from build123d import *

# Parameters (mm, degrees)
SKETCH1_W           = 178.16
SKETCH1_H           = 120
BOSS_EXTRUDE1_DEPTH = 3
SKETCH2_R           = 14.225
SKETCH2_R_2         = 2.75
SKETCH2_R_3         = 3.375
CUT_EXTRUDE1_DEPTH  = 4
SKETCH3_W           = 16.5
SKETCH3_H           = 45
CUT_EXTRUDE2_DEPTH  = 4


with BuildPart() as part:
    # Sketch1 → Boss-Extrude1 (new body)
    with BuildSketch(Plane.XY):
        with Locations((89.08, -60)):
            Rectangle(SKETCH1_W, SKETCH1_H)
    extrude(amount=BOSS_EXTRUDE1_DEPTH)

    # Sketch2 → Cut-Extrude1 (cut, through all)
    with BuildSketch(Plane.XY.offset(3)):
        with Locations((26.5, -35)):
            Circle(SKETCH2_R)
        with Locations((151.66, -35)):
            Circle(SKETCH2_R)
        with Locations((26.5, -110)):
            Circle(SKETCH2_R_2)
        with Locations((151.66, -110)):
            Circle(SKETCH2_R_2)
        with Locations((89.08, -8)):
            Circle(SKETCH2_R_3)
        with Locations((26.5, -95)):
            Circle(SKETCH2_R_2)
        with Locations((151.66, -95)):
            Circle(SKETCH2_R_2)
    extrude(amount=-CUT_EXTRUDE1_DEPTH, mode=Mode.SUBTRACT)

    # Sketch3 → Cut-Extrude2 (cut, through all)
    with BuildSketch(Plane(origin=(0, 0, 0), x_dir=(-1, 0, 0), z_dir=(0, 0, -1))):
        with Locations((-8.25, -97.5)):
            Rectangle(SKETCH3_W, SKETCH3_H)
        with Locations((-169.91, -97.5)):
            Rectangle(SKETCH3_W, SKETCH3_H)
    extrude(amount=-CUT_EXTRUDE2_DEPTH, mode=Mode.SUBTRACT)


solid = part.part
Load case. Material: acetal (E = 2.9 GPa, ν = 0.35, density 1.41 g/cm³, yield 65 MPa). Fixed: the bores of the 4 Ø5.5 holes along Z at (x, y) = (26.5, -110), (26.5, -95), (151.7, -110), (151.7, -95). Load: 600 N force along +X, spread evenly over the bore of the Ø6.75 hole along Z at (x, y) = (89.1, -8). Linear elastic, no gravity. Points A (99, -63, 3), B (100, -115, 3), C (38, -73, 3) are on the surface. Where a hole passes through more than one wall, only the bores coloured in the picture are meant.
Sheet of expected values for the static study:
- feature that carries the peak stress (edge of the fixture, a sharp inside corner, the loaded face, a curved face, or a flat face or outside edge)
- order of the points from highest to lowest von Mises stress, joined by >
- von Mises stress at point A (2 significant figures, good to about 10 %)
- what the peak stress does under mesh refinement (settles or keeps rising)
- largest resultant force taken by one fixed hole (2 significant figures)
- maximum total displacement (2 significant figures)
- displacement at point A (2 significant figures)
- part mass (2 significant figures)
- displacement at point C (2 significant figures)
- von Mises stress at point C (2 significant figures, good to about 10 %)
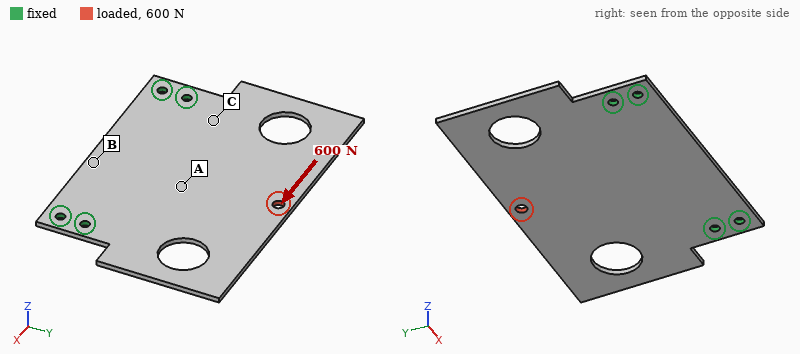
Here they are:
edge of the fixture
C > A > B
2.4 MPa
keeps rising
380 N
0.28 mm
0.077 mm
78 g
0.060 mm
4.6 MPa
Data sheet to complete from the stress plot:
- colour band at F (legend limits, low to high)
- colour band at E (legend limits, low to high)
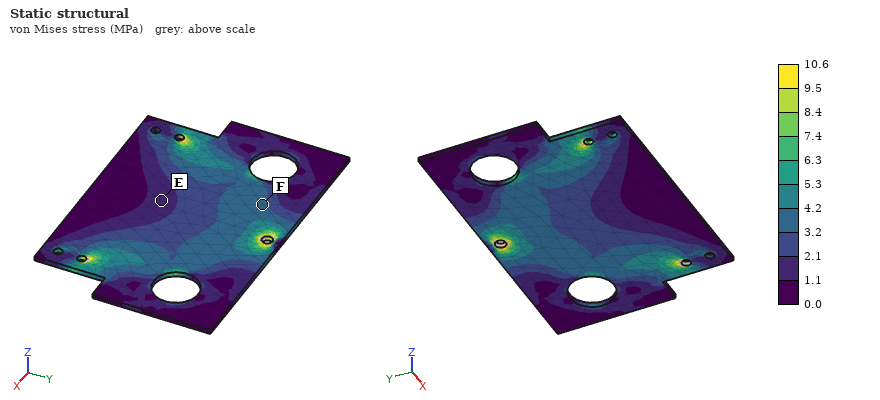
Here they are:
3.2 to 4.2 MPa
1.1 to 2.1 MPa
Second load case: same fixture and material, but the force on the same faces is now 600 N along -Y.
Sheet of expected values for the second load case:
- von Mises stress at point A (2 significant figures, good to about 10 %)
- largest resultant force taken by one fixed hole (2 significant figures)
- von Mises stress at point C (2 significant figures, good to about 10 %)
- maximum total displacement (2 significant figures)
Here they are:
1.6 MPa
210 N
2.8 MPa
0.19 mm
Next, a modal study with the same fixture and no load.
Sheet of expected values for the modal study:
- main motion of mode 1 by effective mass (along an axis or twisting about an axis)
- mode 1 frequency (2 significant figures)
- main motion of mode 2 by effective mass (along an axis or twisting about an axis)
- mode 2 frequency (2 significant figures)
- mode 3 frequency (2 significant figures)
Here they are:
along Z
62 Hz
twisting about Y
110 Hz
200 Hz
